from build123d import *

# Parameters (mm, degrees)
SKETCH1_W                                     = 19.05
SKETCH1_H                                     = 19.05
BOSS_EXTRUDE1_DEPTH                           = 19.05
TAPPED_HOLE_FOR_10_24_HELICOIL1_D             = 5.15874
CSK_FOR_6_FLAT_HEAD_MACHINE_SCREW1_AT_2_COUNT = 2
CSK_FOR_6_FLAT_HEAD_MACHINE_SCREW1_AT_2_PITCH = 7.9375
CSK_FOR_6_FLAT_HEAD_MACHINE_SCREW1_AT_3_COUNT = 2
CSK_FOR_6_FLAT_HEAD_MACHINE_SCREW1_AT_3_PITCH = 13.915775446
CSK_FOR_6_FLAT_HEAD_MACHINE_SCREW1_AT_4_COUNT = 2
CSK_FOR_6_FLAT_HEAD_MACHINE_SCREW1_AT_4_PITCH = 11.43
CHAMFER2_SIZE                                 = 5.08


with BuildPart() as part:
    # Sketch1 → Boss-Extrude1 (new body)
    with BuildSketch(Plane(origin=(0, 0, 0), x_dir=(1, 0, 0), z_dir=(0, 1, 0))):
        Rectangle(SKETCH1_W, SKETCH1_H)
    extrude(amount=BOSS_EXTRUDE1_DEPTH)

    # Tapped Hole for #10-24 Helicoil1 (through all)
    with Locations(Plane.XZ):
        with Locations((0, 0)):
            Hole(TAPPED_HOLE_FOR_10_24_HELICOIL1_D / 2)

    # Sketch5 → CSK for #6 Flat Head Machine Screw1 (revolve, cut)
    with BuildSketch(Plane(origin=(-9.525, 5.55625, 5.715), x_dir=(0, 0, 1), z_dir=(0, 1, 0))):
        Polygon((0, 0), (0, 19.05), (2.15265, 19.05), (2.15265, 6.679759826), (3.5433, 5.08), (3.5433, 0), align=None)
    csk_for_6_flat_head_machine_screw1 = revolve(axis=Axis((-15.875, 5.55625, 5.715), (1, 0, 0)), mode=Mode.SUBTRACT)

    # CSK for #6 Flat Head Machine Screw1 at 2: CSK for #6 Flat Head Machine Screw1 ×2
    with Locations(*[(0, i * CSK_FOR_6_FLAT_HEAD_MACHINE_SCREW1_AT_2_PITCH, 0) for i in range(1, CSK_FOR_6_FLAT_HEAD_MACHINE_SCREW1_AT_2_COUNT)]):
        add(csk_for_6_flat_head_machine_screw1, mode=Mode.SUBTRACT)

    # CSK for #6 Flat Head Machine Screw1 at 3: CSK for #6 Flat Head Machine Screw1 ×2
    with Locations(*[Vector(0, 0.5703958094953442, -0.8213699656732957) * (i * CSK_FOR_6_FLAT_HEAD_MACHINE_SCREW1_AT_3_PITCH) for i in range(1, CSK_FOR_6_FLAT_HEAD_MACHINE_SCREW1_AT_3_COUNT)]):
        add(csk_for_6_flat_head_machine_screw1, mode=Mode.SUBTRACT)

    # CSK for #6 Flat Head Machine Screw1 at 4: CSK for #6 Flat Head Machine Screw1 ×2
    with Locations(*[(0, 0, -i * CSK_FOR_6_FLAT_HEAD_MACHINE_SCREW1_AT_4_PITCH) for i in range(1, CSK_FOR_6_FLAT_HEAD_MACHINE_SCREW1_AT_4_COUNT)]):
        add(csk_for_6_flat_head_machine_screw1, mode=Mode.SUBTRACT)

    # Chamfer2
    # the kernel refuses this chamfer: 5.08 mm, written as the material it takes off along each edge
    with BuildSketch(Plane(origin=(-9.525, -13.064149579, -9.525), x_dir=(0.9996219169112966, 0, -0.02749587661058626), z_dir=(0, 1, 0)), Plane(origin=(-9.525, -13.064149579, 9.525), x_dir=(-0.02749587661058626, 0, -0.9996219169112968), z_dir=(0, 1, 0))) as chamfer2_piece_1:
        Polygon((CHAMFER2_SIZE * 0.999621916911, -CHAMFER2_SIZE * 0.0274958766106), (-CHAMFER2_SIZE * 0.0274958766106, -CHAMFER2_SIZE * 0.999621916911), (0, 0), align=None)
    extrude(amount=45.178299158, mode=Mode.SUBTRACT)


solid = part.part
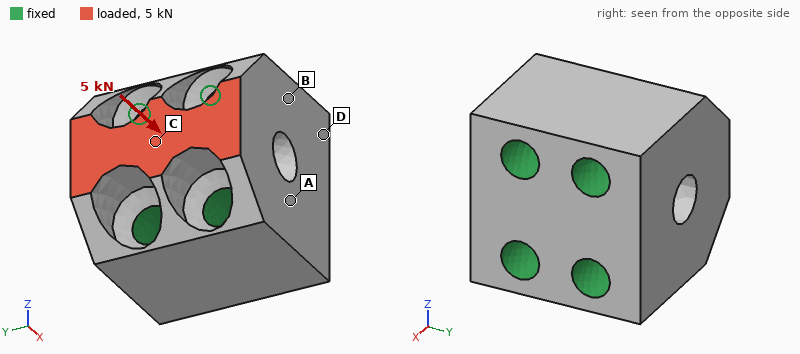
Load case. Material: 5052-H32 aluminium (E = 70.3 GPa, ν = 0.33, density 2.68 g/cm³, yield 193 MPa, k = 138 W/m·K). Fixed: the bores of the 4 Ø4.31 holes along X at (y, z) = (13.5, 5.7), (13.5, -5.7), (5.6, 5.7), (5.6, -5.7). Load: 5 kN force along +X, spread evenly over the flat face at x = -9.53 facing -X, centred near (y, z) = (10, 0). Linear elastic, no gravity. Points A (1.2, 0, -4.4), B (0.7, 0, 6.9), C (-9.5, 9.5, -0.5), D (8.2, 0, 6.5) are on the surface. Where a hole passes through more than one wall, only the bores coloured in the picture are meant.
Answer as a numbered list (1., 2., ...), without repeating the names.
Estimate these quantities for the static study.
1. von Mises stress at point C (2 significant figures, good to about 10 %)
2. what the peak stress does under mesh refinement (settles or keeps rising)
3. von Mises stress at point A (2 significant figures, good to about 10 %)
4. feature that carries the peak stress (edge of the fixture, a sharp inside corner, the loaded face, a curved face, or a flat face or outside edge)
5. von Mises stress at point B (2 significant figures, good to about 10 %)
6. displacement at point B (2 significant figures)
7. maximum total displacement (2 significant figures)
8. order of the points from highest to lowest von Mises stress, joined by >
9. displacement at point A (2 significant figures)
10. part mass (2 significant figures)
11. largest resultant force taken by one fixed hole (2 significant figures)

1. 44 MPa
2. keeps rising
3. 25 MPa
4. edge of the fixture
5. 15 MPa
6. 1.1 µm
7. 7.1 µm
8. C > A > B > D
9. 1.3 µm
10. 12 g
11. 1.4 kN
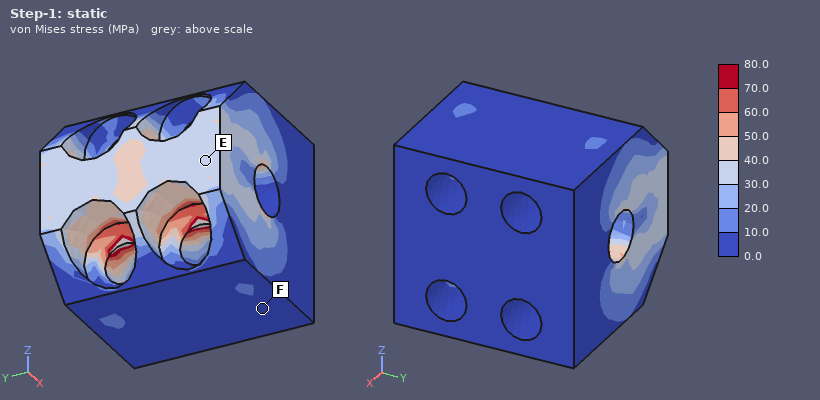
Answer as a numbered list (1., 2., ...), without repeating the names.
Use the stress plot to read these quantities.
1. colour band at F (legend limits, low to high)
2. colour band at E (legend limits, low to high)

1. 0.0 to 10.0 MPa
2. 30.0 to 40.0 MPa
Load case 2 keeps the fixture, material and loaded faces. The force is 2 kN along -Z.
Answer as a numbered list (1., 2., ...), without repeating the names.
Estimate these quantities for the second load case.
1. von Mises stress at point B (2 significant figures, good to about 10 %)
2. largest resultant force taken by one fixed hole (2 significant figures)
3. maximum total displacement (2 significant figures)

1. 9.8 MPa
2. 850 N
3. 8.1 µm
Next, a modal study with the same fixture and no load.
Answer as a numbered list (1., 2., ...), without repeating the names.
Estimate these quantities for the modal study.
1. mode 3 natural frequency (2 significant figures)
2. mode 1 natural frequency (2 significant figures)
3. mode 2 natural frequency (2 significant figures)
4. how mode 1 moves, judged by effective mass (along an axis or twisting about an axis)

1. 87 kHz
2. 62 kHz
3. 85 kHz
4. along Y
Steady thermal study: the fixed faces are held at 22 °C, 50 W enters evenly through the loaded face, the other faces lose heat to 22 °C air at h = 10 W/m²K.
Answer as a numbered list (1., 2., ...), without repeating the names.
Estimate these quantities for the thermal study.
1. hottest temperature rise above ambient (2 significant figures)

1. 23 K
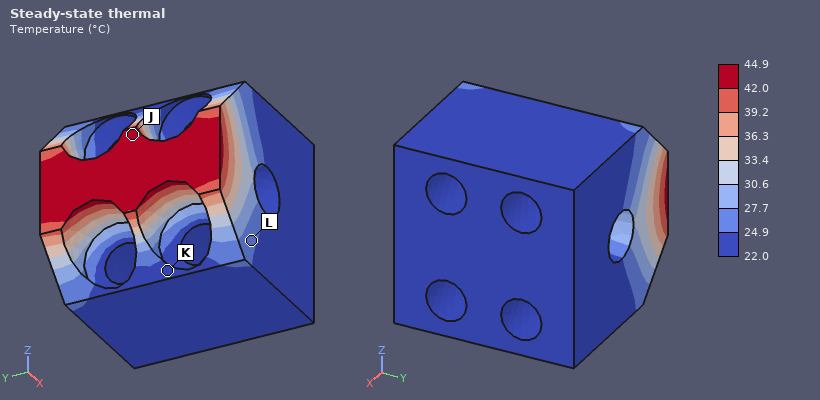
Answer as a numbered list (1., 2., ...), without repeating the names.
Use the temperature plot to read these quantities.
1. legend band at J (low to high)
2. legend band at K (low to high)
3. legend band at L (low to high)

1. 42.0 to 44.9 °C
2. 22.0 to 24.9 °C
3. 24.9 to 27.7 °C
